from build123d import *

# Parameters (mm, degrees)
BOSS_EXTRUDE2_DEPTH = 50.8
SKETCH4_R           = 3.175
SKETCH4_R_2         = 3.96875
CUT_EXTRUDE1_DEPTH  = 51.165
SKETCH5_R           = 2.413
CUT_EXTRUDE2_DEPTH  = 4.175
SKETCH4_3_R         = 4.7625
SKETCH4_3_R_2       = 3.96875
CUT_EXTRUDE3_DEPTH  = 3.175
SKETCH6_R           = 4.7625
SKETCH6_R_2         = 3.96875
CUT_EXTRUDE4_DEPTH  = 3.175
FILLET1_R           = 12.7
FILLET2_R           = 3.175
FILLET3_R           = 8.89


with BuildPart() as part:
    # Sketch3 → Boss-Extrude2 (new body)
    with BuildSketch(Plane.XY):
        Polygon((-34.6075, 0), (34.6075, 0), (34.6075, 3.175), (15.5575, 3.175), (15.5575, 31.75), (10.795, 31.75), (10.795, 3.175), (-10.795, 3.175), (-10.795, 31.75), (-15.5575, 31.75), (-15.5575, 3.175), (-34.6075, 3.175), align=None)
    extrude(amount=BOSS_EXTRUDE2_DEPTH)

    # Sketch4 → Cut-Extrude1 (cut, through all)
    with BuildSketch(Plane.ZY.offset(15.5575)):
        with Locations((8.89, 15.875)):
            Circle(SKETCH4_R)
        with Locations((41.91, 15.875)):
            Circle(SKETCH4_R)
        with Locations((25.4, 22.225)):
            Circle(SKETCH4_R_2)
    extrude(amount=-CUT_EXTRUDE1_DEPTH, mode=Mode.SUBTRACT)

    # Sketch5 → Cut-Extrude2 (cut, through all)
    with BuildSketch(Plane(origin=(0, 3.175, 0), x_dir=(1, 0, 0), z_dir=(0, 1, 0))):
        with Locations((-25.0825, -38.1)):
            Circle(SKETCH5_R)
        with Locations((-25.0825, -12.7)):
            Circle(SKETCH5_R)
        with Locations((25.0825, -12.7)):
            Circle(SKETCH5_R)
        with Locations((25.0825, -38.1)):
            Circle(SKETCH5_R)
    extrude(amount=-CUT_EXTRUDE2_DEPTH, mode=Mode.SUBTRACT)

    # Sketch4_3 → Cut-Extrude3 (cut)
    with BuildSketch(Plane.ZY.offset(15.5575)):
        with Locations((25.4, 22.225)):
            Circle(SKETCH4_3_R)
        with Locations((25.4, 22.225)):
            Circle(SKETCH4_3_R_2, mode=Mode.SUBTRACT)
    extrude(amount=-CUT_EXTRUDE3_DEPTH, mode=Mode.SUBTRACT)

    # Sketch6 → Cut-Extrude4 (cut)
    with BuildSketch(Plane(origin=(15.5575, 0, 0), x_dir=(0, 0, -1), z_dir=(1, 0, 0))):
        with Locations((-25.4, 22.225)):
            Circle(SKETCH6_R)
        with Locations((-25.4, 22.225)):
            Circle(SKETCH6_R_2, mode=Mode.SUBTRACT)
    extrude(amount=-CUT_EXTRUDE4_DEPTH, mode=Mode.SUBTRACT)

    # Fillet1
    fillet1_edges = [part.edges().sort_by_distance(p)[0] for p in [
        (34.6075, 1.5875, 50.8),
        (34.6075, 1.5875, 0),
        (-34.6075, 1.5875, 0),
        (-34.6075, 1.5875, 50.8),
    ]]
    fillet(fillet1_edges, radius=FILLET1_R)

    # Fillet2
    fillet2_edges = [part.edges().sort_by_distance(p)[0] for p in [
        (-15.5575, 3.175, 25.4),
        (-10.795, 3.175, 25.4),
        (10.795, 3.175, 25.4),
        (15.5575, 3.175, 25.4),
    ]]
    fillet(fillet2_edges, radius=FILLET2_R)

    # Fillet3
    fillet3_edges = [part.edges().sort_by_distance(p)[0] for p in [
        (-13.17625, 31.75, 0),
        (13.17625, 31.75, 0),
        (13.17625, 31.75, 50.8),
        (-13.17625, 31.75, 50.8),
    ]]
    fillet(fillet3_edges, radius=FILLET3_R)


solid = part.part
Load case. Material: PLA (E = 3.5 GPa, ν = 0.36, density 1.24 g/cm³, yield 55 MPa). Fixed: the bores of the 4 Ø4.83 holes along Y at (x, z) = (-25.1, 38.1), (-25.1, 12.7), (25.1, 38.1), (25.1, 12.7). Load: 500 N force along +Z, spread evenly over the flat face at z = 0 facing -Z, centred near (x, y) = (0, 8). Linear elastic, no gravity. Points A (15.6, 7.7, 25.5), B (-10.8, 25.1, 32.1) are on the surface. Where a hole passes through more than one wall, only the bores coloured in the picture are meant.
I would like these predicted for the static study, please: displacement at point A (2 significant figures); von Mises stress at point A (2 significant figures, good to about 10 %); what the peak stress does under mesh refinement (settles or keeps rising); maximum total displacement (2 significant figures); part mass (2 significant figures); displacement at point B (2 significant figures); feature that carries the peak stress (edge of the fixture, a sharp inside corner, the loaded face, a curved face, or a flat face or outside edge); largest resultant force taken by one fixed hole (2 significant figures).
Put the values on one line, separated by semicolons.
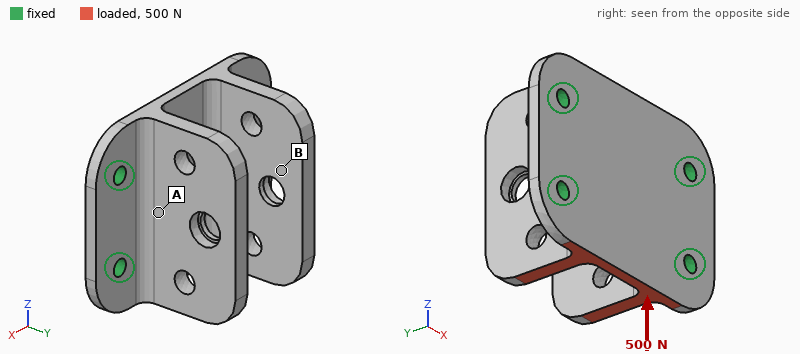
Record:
0.035 mm; 3.0 MPa; keeps rising; 0.14 mm; 29 g; 0.089 mm; edge of the fixture; 150 N
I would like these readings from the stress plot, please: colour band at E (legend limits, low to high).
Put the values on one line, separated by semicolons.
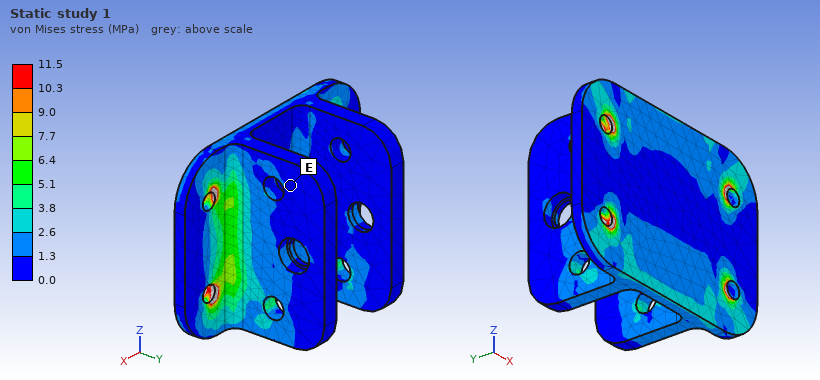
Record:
0.0 to 1.3 MPa
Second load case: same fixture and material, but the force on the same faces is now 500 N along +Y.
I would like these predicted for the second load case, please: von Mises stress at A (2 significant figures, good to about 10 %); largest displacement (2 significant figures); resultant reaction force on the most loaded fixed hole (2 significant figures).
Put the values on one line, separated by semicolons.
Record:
9.8 MPa; 1.0 mm; 350 N
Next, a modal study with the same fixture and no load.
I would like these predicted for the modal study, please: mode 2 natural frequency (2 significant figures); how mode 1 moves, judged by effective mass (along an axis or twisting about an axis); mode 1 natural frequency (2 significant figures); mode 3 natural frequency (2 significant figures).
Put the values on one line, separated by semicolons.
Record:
1400 Hz; along Y; 830 Hz; 1400 Hz
